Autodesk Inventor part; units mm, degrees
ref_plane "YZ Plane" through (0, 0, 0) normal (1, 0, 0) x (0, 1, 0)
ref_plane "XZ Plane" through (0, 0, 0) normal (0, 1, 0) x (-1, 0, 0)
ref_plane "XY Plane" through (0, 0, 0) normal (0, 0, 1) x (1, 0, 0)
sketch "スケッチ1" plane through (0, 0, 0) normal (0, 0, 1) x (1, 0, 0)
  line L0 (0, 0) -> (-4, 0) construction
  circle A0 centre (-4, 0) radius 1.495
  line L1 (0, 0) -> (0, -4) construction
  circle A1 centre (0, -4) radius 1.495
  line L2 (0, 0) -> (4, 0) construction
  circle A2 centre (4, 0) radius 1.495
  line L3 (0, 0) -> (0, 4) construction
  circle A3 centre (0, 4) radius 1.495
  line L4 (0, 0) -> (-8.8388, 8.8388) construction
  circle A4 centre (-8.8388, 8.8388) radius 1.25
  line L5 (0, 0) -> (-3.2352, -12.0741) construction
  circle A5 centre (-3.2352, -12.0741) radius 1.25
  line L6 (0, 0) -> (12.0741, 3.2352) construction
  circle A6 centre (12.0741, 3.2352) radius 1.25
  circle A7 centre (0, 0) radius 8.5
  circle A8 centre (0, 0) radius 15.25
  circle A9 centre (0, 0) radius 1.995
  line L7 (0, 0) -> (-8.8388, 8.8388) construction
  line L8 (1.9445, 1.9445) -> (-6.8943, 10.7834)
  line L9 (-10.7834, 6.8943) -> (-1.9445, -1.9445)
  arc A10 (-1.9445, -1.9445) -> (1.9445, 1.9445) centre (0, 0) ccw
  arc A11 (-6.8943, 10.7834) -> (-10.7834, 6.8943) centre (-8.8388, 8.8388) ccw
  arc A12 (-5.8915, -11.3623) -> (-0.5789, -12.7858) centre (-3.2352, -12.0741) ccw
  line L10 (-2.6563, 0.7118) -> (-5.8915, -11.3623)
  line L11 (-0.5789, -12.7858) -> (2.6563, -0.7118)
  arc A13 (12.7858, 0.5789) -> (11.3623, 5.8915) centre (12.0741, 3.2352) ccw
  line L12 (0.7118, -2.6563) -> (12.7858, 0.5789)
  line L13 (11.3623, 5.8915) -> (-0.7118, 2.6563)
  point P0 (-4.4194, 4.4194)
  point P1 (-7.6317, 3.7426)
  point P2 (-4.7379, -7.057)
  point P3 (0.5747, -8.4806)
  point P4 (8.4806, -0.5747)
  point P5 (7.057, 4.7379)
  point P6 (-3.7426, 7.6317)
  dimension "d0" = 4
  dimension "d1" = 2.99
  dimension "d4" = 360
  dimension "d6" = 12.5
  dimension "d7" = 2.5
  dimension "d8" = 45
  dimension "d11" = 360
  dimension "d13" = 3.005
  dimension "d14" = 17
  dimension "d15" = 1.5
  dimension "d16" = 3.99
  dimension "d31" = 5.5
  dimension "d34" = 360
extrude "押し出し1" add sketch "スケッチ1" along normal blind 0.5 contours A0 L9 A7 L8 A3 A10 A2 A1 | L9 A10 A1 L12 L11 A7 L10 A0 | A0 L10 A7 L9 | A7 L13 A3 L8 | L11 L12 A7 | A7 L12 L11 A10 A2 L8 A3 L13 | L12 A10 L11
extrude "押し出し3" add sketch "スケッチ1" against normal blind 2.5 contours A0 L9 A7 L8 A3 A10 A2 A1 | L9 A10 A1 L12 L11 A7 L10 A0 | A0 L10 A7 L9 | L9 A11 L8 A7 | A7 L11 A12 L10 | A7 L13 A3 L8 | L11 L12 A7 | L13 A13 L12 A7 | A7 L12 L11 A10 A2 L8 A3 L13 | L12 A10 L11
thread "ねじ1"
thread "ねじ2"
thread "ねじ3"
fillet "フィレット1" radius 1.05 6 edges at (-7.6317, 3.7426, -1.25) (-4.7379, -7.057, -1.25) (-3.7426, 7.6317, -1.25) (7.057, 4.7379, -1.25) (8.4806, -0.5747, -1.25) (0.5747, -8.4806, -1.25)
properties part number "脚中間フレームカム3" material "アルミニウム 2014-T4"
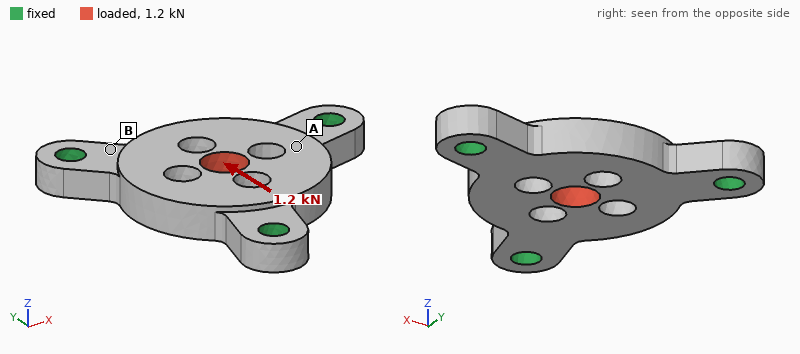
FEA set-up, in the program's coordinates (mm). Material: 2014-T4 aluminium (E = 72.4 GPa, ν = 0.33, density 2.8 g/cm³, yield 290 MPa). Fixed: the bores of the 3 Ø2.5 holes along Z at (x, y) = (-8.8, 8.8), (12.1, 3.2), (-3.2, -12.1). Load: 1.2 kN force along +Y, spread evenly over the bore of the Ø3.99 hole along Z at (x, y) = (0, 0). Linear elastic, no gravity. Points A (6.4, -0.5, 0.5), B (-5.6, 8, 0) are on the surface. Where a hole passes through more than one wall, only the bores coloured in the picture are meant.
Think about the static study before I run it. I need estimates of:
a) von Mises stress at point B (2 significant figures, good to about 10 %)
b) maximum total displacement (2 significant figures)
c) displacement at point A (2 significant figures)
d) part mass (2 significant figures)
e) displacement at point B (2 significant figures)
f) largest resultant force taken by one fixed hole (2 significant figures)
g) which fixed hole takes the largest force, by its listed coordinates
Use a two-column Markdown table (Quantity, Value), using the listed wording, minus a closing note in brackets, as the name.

| Quantity | Value |
|---|---|
| von Mises stress at point B | 37 MPa |
| maximum total displacement | 14 µm |
| displacement at point A | 7.4 µm |
| part mass | 2.2 g |
| displacement at point B | 2.7 µm |
| largest resultant force taken by one fixed hole | 570 N |
| which fixed hole takes the largest force, by its listed coordinates | (-3.2, -12.1) |
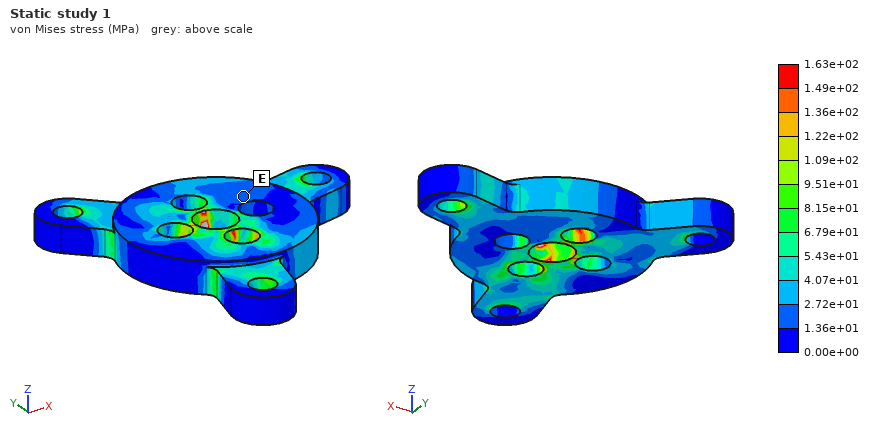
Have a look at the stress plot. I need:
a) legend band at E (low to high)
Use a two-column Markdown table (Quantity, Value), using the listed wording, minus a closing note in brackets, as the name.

| Quantity | Value |
|---|---|
| legend band at E | 1.36e+01 to 2.72e+01 MPa |
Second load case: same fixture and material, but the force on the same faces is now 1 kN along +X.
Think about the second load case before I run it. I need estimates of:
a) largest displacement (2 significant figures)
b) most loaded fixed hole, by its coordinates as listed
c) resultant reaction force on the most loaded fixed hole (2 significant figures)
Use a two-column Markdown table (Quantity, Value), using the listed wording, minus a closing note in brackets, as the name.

| Quantity | Value |
|---|---|
| largest displacement | 12 µm |
| most loaded fixed hole, by its coordinates as listed | (12.1, 3.2) |
| resultant reaction force on the most loaded fixed hole | 480 N |
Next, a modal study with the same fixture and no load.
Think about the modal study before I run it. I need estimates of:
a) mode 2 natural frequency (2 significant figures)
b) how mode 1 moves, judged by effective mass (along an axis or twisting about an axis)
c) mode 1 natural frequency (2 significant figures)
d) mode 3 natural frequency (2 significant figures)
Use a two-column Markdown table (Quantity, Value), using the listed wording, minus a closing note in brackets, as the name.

| Quantity | Value |
|---|---|
| mode 2 natural frequency | 33 kHz |
| how mode 1 moves, judged by effective mass | along Z |
| mode 1 natural frequency | 25 kHz |
| mode 3 natural frequency | 33 kHz |
